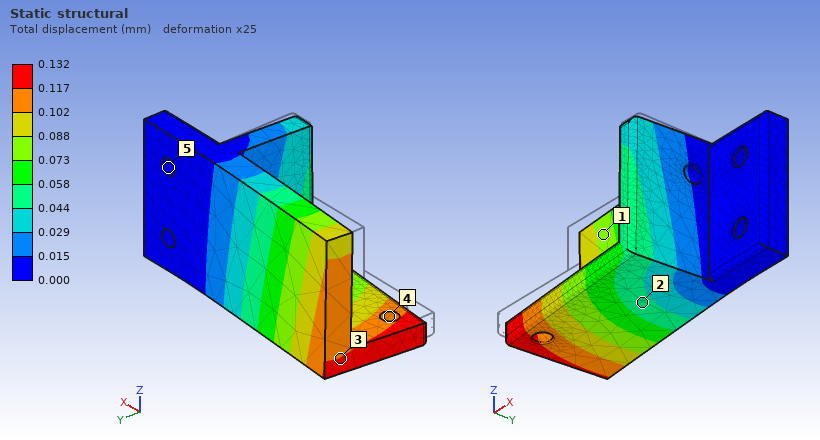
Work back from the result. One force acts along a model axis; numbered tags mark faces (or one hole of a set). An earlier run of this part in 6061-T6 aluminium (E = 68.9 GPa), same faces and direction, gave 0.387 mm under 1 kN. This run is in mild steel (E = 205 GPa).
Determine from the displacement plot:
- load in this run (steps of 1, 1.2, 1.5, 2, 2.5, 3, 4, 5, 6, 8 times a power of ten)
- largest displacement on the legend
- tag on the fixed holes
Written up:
1 kN
0.132 mm
5
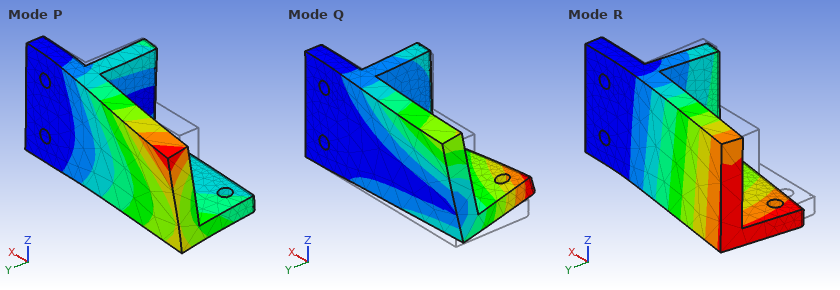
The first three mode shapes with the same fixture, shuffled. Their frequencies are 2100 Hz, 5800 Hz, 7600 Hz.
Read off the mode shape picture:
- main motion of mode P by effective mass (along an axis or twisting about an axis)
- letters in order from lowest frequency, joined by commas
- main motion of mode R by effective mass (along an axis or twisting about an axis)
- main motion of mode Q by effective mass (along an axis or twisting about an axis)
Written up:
along Z
R, Q, P
along Y
along Z
